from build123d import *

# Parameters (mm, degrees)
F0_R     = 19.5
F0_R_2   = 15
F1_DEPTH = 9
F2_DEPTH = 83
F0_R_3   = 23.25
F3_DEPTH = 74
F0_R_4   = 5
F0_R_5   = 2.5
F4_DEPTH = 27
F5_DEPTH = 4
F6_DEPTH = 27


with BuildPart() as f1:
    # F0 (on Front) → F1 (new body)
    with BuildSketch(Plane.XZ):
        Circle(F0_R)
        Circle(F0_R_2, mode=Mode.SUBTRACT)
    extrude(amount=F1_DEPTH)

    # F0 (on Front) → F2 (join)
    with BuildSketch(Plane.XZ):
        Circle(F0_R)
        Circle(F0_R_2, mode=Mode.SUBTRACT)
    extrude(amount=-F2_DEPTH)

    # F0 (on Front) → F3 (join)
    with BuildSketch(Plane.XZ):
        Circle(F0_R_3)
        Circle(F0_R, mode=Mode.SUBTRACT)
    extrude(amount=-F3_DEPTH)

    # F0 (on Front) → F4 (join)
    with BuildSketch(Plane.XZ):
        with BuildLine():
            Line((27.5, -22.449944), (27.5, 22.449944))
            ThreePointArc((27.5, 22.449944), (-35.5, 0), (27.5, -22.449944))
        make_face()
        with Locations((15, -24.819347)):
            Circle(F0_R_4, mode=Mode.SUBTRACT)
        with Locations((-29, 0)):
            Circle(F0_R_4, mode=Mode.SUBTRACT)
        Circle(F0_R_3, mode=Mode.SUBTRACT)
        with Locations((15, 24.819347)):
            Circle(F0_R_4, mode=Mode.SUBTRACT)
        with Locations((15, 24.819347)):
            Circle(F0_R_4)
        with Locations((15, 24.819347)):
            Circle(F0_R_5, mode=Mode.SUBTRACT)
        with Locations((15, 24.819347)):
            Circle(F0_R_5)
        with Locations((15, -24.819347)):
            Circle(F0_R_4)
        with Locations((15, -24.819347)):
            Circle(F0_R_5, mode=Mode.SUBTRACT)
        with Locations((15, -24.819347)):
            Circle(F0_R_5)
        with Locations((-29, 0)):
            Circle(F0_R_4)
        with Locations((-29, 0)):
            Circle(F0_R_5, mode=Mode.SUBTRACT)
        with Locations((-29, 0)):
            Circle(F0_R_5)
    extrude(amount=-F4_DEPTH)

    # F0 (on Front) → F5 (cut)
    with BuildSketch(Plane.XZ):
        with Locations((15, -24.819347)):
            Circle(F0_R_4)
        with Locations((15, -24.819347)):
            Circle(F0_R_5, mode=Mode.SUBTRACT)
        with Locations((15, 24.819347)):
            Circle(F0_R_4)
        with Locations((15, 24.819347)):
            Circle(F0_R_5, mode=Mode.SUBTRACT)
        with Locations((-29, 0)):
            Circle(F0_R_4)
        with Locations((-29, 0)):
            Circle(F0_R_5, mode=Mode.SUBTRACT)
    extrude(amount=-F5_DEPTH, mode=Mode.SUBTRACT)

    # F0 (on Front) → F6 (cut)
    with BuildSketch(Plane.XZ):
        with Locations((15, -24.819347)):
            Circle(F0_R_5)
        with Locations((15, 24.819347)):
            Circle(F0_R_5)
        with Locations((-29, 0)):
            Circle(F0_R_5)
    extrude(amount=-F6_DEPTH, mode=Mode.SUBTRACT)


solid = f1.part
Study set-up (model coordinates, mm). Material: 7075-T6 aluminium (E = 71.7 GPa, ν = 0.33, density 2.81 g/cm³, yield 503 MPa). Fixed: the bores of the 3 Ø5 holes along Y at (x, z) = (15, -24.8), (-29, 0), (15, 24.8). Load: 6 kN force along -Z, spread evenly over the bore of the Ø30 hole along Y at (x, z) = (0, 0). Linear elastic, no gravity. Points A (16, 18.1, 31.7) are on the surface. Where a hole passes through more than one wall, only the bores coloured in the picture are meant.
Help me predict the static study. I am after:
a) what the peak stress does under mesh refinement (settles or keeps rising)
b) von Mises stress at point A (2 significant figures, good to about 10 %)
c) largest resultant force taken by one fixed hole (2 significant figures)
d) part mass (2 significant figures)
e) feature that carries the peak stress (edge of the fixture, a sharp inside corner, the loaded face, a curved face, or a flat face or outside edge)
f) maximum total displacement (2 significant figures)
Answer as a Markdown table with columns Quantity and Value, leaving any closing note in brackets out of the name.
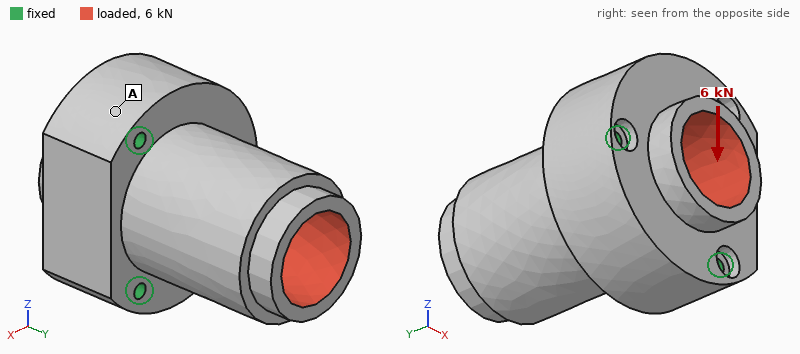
| Quantity | Value |
|---|---|
| what the peak stress does under mesh refinement | keeps rising |
| von Mises stress at point A | 3.7 MPa |
| largest resultant force taken by one fixed hole | 2.8 kN |
| part mass | 380 g |
| feature that carries the peak stress | edge of the fixture |
| maximum total displacement | 23 µm |
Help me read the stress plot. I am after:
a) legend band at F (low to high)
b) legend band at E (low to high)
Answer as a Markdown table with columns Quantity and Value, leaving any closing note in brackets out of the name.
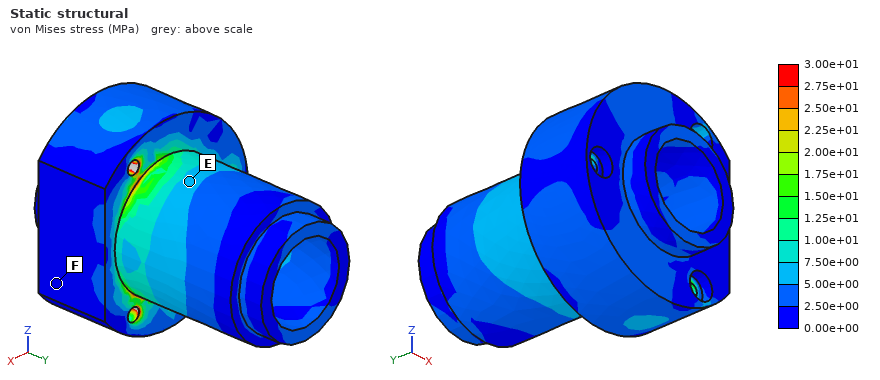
| Quantity | Value |
|---|---|
| legend band at F | 0.00e+00 to 2.50e+00 MPa |
| legend band at E | 5.00e+00 to 7.50e+00 MPa |
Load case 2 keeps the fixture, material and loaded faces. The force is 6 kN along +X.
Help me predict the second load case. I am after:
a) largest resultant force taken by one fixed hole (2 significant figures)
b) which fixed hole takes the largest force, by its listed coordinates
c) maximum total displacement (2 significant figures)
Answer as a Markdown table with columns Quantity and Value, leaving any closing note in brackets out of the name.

| Quantity | Value |
|---|---|
| largest resultant force taken by one fixed hole | 3.1 kN |
| which fixed hole takes the largest force, by its listed coordinates | (-29, 0) |
| maximum total displacement | 23 µm |
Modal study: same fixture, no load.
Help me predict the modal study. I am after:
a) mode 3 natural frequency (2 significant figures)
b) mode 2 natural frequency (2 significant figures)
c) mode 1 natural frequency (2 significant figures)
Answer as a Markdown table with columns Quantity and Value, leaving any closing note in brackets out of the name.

| Quantity | Value |
|---|---|
| mode 3 natural frequency | 14 kHz |
| mode 2 natural frequency | 6600 Hz |
| mode 1 natural frequency | 6600 Hz |
